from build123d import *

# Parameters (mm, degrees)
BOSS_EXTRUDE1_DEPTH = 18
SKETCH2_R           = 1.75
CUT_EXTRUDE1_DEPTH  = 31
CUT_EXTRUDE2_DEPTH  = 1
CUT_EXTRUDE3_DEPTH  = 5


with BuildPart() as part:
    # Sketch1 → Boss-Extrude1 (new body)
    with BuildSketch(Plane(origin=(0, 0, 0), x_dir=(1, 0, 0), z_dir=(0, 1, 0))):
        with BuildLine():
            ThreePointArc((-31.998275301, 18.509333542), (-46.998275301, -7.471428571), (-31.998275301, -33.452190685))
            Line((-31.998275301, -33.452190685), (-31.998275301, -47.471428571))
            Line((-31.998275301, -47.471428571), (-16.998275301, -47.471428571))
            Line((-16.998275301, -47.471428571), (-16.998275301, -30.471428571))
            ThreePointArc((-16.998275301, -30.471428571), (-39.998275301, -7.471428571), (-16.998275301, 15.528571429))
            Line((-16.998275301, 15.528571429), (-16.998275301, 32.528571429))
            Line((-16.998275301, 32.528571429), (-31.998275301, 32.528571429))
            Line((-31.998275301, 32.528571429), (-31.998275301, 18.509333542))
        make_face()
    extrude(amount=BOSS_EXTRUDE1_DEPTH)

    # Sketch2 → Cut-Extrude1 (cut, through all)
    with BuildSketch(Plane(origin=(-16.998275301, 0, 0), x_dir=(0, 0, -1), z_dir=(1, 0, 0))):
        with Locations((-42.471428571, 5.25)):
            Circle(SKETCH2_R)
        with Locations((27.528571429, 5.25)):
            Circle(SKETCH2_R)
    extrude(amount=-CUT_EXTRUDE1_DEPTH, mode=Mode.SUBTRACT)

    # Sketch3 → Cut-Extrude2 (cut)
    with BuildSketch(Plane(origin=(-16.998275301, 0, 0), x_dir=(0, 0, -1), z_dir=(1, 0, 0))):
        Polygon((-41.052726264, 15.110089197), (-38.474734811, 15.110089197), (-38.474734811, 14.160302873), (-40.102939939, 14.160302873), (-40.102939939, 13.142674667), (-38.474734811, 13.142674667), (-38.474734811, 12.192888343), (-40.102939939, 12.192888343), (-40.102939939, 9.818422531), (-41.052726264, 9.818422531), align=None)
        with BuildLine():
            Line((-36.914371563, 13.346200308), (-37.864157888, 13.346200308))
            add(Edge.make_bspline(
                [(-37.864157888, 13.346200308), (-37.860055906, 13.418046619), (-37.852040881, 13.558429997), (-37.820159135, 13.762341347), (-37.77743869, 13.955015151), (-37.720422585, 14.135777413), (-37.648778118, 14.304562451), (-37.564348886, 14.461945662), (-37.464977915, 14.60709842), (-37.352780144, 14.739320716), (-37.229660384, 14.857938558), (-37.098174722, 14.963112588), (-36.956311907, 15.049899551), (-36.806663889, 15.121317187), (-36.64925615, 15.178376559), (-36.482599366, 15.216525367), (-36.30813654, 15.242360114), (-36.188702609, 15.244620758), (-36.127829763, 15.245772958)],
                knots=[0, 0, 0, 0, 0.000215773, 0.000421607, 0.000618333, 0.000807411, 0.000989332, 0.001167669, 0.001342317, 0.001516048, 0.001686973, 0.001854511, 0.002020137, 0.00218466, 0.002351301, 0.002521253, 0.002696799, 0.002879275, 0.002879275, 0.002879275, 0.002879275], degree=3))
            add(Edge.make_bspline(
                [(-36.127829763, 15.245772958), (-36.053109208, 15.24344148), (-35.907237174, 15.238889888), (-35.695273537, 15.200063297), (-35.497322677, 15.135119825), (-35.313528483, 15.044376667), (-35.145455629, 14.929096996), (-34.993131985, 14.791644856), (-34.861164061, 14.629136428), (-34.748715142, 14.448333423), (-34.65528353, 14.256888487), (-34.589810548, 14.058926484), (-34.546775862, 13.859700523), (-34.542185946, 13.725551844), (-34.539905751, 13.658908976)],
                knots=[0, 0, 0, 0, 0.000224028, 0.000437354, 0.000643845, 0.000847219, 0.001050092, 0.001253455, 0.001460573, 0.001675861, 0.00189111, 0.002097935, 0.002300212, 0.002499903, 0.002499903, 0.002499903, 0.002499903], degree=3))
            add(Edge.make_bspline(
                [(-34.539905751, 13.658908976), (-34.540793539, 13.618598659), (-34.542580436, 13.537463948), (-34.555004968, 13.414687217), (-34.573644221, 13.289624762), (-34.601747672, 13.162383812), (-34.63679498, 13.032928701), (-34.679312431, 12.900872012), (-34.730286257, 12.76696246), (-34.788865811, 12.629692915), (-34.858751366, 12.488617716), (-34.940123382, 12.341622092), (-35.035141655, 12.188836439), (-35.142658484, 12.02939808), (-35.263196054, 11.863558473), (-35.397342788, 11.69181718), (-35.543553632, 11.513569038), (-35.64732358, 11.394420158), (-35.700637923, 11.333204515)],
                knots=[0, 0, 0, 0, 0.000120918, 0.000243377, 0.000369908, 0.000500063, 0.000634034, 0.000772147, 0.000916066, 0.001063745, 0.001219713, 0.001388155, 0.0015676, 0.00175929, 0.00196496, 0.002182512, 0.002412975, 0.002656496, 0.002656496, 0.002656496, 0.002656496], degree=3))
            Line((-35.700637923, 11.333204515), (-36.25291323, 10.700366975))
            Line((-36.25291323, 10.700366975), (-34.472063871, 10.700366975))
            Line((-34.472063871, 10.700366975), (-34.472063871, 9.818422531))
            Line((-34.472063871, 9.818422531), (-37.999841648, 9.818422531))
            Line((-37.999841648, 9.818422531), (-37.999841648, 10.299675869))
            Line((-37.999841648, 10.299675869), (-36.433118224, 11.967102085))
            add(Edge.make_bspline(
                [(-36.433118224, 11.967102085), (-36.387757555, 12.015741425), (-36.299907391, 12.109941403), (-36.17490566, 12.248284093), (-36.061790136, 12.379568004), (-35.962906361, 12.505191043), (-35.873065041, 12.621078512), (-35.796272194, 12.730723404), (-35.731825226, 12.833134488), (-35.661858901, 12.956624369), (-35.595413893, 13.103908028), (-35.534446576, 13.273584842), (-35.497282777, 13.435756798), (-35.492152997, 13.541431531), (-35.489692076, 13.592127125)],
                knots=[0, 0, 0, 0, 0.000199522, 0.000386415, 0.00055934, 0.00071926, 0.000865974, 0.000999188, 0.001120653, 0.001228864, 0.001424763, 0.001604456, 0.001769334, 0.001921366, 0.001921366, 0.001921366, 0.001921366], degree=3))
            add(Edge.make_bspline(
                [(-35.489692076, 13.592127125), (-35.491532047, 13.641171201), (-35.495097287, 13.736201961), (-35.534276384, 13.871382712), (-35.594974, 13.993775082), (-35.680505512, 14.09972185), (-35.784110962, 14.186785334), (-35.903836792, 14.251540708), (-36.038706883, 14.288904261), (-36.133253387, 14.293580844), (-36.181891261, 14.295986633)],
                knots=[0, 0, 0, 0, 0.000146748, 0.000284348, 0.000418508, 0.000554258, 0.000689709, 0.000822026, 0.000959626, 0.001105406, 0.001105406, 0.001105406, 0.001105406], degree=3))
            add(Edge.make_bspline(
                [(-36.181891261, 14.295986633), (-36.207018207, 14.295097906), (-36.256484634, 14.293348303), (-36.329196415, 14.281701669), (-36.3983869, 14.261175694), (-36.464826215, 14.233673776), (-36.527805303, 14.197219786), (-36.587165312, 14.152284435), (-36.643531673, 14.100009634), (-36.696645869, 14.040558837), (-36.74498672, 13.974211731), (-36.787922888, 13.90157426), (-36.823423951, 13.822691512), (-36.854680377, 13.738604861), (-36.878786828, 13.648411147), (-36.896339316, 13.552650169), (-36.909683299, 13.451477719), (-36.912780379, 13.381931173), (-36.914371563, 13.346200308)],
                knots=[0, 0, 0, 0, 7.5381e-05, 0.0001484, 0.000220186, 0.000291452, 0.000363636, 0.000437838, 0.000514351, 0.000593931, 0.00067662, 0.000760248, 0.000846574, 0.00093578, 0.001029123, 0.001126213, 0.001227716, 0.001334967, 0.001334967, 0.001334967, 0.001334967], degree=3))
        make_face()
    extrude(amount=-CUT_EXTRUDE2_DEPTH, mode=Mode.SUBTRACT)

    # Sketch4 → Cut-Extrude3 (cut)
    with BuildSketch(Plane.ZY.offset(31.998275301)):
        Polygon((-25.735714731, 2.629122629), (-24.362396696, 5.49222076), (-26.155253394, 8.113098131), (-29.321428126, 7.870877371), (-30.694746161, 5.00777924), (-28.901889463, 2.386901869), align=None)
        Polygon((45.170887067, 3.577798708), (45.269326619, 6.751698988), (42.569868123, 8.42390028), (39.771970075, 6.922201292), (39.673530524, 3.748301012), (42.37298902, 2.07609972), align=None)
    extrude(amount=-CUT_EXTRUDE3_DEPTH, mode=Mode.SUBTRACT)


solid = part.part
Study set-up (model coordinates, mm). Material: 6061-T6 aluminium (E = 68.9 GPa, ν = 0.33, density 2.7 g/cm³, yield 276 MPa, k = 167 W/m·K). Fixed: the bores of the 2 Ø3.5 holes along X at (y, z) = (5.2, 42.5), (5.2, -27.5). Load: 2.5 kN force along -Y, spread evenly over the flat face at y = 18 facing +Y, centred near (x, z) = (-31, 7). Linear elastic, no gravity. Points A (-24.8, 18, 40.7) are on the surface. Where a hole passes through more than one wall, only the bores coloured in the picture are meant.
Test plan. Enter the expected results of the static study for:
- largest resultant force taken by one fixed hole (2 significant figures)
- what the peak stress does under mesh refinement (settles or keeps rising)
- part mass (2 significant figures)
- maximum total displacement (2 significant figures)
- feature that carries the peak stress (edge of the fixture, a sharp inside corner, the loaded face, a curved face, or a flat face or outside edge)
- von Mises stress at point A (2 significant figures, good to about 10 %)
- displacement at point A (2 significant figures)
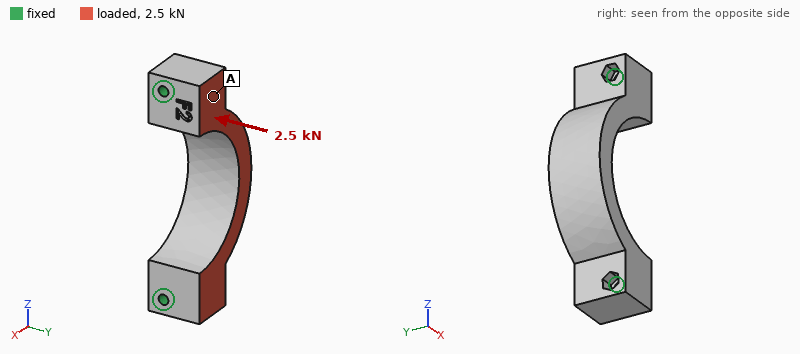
1.3 kN
keeps rising
44 g
60 µm
edge of the fixture
11 MPa
15 µm
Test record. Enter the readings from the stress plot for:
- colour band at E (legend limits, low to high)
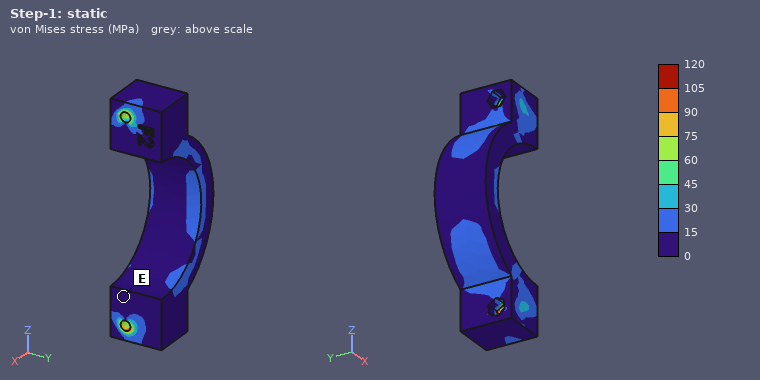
0 to 15 MPa
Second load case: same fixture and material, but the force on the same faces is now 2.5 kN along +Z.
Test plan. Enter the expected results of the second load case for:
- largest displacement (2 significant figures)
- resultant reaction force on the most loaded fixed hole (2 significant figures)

16 µm
1.3 kN
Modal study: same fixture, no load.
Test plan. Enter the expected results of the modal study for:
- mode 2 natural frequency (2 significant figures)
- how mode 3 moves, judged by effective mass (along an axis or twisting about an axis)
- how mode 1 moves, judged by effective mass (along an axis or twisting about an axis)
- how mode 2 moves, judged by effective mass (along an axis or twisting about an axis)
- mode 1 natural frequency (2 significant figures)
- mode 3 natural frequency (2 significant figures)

12 kHz
along X
along Y
along Z
6000 Hz
17 kHz
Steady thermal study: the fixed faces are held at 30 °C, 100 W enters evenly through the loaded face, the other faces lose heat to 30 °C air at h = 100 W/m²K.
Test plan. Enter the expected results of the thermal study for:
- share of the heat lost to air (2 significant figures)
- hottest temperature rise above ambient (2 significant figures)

8.1 %
32 K
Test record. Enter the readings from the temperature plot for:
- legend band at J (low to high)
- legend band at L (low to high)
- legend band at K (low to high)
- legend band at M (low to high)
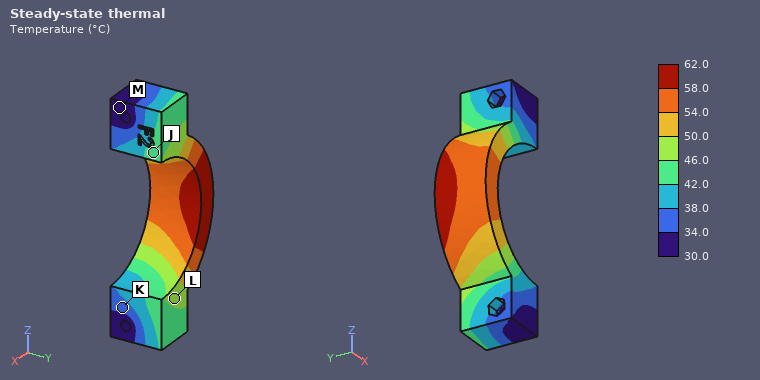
42.0 to 46.0 °C
46.0 to 50.0 °C
34.0 to 38.0 °C
30.0 to 34.0 °C
